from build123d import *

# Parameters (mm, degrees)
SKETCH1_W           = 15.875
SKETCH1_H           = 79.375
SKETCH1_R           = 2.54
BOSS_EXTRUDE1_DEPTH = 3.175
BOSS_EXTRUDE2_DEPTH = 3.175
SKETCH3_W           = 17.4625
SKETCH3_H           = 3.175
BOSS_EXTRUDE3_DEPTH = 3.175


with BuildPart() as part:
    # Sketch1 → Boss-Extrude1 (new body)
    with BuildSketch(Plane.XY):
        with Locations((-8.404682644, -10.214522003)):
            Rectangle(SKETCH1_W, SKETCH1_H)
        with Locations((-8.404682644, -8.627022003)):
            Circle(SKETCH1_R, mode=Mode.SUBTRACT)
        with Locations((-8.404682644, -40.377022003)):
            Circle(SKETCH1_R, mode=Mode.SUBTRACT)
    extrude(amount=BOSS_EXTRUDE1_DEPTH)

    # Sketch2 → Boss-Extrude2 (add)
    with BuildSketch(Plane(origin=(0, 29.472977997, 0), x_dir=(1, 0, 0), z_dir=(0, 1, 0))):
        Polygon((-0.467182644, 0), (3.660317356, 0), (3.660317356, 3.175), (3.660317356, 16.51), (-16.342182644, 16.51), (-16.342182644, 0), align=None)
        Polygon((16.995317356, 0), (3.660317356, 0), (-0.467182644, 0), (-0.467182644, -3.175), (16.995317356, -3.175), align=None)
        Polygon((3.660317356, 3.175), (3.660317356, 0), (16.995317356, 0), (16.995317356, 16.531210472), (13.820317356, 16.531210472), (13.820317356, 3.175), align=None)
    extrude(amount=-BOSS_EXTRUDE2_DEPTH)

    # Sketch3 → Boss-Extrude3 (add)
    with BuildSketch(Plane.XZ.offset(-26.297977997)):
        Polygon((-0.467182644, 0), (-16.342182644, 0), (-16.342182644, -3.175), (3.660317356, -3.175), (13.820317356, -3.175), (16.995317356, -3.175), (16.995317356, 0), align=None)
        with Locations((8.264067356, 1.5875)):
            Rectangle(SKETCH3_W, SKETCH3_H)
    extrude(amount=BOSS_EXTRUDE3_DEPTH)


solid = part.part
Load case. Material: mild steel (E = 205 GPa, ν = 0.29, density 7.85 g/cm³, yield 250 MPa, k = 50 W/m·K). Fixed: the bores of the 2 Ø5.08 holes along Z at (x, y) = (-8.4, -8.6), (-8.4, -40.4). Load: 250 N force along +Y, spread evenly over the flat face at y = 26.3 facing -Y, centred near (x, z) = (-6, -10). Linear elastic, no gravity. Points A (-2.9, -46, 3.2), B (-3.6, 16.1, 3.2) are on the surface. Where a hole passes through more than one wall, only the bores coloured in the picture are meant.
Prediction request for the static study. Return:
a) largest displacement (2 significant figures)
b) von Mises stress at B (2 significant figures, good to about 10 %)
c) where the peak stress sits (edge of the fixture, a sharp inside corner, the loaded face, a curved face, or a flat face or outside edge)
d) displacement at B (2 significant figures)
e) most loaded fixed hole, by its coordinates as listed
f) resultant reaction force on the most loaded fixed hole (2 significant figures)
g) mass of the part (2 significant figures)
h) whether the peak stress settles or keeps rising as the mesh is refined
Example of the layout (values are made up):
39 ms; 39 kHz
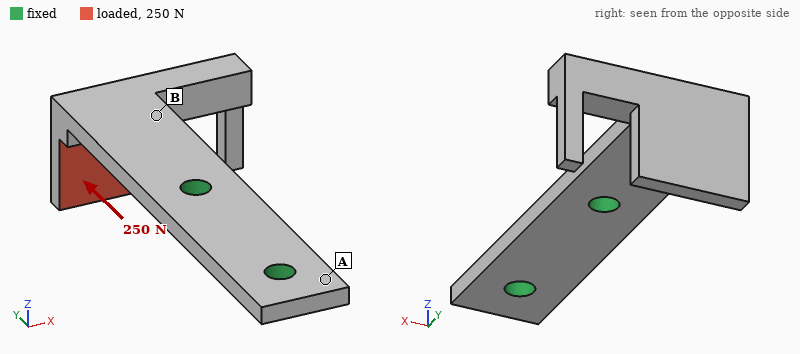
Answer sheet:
0.30 mm; 99 MPa; edge of the fixture; 0.090 mm; (-8.4, -8.6); 240 N; 46 g; keeps rising
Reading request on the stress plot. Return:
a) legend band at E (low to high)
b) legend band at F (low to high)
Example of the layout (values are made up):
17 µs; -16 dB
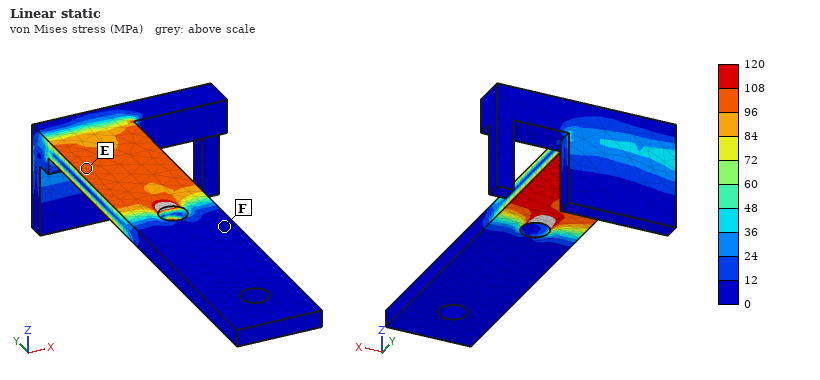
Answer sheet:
96 to 108 MPa; 0 to 12 MPa
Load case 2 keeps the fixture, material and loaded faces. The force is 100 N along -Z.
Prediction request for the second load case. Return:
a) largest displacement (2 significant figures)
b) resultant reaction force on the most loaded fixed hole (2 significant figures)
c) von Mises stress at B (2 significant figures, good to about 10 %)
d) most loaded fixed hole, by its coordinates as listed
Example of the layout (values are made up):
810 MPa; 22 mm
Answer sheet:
0.21 mm; 100 N; 39 MPa; (-8.4, -8.6)
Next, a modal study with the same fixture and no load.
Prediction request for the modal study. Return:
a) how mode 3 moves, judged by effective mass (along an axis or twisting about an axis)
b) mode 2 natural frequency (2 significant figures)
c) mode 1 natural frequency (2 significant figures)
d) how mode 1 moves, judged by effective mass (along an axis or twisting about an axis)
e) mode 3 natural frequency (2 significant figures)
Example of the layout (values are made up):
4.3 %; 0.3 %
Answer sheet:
along X; 1800 Hz; 830 Hz; along Z; 3500 Hz
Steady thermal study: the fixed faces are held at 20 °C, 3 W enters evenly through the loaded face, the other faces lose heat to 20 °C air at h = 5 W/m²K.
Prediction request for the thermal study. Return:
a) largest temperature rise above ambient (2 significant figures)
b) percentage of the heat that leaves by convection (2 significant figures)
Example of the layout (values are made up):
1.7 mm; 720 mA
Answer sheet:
44 K; 12 %
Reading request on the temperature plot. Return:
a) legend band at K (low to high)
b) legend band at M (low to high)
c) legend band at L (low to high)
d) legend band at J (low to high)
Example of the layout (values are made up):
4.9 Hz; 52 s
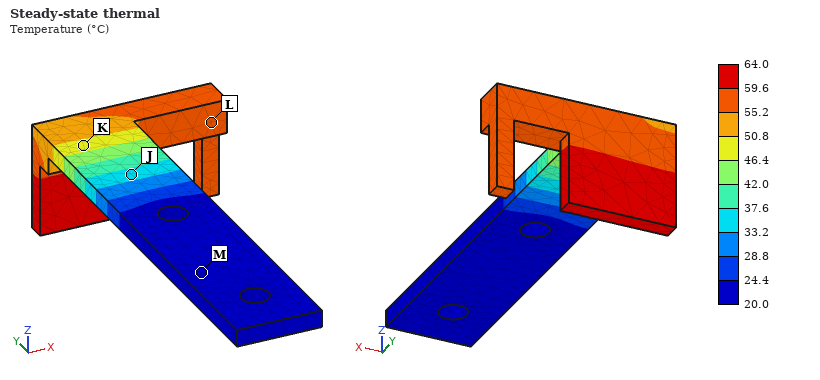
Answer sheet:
46.4 to 50.8 °C; 20.0 to 24.4 °C; 55.2 to 59.6 °C; 33.2 to 37.6 °C
